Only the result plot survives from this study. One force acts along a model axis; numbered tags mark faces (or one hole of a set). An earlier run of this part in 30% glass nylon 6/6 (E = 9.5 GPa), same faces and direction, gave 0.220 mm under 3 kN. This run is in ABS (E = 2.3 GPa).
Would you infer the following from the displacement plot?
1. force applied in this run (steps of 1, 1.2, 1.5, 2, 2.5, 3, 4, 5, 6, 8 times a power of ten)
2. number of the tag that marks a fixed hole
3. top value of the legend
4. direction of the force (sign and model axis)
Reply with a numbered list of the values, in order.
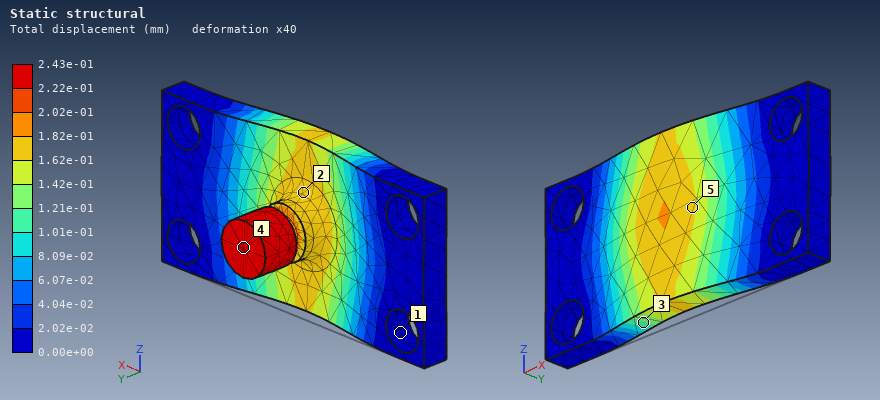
1. 800 N
2. 1
3. 2.43e-01 mm
4. -Y
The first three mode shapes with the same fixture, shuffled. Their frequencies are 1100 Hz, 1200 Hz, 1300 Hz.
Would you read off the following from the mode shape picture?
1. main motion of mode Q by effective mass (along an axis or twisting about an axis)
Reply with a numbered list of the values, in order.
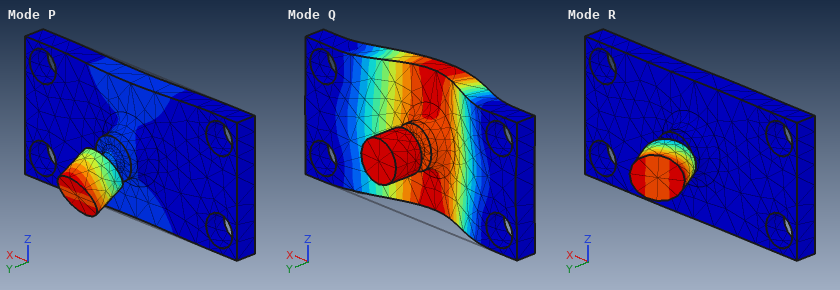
1. along Y
